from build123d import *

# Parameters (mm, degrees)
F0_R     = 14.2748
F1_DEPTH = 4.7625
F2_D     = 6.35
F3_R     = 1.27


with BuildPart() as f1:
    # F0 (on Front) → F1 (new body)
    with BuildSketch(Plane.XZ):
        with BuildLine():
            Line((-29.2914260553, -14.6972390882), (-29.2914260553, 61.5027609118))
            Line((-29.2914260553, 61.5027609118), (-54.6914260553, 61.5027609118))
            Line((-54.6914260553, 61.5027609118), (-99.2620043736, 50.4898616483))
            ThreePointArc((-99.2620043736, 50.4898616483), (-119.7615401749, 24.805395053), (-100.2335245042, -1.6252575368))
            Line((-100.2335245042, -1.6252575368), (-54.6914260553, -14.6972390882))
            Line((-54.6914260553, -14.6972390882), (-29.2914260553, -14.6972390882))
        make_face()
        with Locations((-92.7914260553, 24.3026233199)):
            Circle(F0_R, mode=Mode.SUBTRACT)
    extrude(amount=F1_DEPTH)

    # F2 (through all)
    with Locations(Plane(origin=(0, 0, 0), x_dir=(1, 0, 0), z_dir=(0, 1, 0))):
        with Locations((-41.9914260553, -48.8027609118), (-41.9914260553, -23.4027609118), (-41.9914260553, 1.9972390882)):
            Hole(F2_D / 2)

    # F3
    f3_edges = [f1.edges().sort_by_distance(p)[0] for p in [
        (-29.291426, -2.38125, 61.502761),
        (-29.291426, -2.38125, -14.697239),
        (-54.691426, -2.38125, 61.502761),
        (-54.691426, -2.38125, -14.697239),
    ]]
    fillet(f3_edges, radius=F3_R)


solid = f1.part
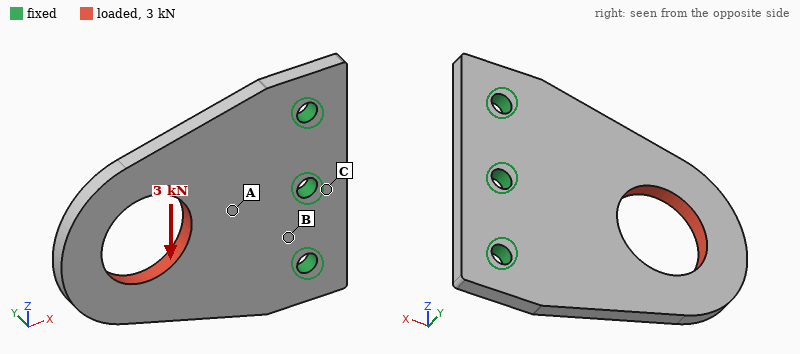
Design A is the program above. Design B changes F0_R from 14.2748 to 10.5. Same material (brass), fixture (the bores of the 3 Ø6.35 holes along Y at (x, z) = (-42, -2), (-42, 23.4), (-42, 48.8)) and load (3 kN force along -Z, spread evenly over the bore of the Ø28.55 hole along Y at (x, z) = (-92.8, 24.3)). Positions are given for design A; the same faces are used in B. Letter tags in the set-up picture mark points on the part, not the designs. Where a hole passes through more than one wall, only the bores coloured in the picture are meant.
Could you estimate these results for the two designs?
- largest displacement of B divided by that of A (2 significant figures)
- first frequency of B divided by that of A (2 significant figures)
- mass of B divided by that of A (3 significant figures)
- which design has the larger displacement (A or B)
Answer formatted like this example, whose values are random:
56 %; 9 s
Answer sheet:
0.77; 0.96; 1.06; A
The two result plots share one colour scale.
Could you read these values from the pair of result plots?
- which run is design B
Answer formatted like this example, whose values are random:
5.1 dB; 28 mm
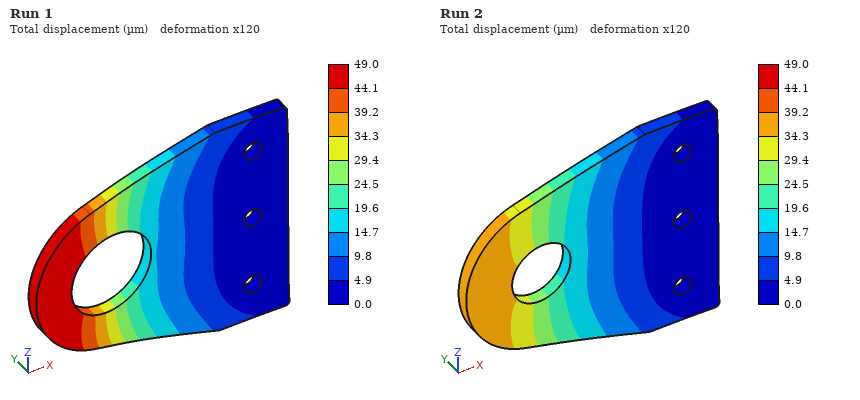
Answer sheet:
Run 2
